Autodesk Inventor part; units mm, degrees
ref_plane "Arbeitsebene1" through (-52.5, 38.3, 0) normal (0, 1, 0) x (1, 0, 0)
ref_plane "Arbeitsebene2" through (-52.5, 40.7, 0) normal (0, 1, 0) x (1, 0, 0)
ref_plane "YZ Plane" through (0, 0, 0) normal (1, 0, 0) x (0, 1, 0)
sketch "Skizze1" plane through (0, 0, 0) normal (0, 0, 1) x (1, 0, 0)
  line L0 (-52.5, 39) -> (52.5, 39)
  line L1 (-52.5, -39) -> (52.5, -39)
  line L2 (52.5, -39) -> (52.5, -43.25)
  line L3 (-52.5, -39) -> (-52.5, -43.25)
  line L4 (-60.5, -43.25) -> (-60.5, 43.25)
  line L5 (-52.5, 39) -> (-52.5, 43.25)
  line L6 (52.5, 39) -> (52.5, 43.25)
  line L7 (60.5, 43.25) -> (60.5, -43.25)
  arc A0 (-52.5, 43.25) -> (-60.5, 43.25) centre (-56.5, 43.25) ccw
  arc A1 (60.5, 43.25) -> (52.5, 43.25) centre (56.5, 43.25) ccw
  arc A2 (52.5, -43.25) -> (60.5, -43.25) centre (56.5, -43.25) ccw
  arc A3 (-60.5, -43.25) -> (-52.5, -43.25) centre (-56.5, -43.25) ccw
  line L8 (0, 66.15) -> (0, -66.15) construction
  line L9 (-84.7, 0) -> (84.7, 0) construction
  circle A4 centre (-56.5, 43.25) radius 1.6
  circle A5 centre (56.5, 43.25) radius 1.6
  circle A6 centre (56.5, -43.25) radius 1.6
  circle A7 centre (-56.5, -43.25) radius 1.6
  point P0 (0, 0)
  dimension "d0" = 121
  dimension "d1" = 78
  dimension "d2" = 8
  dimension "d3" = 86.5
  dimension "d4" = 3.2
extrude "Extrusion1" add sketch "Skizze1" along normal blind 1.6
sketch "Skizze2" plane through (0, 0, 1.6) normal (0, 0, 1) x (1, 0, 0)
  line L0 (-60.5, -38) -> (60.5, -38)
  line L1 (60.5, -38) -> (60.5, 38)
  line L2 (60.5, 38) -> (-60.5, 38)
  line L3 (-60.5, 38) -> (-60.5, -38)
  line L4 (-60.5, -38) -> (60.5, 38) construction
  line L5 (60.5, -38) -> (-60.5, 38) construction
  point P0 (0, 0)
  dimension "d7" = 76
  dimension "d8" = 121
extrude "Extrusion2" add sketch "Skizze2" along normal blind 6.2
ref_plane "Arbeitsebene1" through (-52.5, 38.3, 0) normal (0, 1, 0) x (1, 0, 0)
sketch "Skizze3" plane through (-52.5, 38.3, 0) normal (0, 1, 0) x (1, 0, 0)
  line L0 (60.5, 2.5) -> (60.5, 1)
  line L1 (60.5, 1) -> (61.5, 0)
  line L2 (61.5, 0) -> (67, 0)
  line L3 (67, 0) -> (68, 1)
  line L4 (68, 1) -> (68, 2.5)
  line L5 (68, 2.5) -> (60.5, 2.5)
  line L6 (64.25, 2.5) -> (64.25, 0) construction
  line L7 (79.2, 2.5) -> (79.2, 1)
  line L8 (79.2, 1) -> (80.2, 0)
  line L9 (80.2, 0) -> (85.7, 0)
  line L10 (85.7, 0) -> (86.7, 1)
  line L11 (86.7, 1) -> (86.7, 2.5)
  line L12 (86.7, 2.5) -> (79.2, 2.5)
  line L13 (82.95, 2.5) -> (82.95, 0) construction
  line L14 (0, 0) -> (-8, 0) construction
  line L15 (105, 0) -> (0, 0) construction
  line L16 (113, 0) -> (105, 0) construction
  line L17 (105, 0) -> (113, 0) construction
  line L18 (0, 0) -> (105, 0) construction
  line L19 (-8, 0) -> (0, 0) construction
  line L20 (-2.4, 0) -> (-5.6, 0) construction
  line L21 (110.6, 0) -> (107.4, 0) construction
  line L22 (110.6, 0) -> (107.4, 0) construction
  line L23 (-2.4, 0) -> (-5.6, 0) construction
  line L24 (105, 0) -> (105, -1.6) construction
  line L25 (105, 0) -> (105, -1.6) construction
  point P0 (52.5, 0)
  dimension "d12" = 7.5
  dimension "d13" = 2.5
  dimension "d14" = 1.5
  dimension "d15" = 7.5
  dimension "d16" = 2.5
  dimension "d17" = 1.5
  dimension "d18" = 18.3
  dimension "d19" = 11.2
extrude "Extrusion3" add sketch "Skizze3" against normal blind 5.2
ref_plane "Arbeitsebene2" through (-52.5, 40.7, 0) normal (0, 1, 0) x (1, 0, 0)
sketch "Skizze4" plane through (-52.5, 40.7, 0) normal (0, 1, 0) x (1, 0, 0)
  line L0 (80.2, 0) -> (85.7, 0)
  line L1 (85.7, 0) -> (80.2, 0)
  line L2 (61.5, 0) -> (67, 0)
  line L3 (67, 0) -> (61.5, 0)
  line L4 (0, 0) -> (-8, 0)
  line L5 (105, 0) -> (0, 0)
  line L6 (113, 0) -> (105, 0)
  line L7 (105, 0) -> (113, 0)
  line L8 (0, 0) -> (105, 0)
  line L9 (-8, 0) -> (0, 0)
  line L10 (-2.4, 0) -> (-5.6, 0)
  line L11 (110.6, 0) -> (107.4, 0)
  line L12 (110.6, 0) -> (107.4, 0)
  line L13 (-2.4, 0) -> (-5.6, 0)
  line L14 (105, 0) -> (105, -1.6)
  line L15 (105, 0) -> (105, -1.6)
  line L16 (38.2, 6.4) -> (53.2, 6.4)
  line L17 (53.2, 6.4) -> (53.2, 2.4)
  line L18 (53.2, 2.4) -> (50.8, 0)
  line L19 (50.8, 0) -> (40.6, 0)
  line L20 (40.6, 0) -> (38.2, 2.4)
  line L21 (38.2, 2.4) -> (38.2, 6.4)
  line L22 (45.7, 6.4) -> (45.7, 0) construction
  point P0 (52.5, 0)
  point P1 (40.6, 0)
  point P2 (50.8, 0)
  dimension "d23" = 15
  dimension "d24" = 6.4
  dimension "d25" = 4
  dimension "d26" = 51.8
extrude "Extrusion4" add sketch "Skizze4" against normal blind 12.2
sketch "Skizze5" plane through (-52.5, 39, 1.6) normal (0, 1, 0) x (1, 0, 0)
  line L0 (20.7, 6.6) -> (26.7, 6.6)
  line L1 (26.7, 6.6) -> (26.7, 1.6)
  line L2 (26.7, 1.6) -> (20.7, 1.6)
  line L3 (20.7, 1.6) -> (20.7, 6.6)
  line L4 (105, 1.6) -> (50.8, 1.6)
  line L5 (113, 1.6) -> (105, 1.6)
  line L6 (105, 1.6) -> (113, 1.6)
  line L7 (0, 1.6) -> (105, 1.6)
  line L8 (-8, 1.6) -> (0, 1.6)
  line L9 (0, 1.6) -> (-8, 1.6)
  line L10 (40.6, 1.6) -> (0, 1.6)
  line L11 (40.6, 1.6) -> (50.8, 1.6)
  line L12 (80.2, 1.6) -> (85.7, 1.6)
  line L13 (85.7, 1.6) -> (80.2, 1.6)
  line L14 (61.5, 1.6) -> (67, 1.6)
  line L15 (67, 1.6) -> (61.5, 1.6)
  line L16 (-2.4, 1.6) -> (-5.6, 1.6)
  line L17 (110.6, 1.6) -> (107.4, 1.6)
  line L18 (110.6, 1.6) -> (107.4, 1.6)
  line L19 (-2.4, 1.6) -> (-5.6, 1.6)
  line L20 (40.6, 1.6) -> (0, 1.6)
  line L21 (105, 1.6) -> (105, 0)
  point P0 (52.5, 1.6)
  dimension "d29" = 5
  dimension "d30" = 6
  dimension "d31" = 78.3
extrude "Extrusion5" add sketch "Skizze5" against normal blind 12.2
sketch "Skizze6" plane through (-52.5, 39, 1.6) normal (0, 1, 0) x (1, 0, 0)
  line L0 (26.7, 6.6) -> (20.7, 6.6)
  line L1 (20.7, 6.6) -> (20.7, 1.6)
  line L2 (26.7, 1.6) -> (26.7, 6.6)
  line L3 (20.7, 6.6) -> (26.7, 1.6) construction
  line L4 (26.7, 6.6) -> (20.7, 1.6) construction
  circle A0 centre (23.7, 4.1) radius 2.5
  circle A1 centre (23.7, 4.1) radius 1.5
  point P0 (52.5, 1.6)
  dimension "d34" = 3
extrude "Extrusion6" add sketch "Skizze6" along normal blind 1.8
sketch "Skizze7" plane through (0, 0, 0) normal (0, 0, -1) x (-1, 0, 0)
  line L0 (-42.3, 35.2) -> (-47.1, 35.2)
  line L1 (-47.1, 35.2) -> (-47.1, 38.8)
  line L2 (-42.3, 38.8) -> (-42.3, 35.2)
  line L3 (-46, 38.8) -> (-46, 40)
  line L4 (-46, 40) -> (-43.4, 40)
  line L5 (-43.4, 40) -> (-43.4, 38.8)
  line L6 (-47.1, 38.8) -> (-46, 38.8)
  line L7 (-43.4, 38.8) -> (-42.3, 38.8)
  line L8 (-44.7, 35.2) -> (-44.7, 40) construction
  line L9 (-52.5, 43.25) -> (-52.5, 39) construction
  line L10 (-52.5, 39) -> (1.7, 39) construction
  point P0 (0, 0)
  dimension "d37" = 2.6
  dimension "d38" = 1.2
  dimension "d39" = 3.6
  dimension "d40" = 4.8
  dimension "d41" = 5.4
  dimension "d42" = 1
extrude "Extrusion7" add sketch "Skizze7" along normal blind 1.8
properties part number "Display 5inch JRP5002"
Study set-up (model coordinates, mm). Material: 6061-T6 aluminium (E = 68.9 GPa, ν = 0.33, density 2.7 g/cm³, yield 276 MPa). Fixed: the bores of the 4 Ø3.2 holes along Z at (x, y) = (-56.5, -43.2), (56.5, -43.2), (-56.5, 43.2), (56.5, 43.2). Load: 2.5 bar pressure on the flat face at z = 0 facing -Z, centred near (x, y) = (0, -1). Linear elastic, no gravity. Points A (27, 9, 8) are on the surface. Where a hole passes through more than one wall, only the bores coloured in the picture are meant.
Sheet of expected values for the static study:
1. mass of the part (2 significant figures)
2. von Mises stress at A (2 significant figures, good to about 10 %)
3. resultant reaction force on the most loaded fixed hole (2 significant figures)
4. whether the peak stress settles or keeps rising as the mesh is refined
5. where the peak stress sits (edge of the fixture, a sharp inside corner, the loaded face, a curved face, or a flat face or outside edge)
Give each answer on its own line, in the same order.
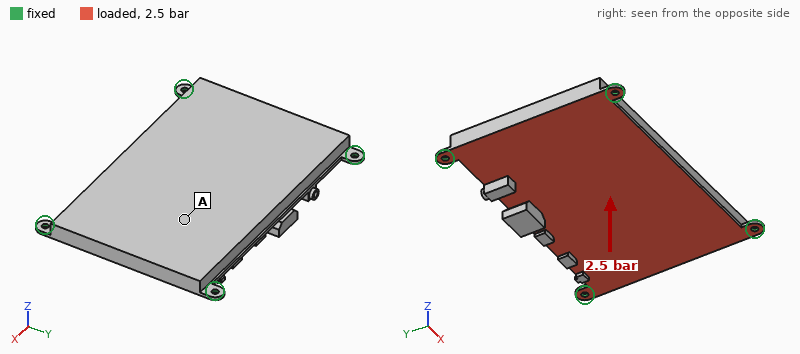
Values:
200 g
22 MPa
1.1 kN
keeps rising
edge of the fixture
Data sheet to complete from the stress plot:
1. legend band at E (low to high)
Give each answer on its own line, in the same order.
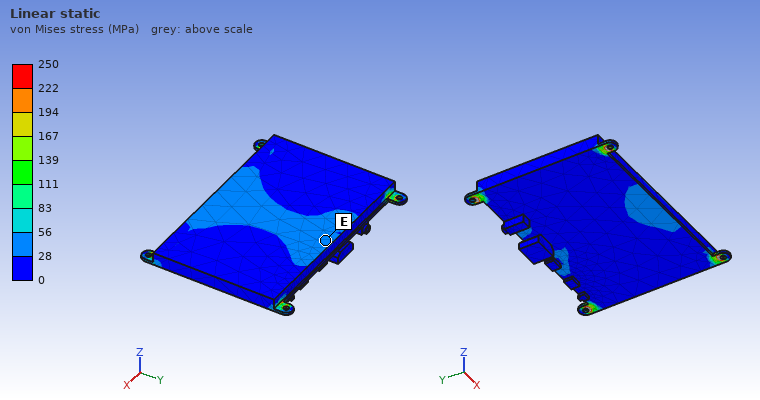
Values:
28 to 56 MPa
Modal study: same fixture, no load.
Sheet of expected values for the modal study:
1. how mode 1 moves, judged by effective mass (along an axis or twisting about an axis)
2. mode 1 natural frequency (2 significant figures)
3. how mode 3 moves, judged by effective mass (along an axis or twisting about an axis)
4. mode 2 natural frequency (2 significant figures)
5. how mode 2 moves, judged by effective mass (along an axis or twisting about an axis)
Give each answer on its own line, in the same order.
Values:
along Z
1300 Hz
twisting about Y
2600 Hz
twisting about X
